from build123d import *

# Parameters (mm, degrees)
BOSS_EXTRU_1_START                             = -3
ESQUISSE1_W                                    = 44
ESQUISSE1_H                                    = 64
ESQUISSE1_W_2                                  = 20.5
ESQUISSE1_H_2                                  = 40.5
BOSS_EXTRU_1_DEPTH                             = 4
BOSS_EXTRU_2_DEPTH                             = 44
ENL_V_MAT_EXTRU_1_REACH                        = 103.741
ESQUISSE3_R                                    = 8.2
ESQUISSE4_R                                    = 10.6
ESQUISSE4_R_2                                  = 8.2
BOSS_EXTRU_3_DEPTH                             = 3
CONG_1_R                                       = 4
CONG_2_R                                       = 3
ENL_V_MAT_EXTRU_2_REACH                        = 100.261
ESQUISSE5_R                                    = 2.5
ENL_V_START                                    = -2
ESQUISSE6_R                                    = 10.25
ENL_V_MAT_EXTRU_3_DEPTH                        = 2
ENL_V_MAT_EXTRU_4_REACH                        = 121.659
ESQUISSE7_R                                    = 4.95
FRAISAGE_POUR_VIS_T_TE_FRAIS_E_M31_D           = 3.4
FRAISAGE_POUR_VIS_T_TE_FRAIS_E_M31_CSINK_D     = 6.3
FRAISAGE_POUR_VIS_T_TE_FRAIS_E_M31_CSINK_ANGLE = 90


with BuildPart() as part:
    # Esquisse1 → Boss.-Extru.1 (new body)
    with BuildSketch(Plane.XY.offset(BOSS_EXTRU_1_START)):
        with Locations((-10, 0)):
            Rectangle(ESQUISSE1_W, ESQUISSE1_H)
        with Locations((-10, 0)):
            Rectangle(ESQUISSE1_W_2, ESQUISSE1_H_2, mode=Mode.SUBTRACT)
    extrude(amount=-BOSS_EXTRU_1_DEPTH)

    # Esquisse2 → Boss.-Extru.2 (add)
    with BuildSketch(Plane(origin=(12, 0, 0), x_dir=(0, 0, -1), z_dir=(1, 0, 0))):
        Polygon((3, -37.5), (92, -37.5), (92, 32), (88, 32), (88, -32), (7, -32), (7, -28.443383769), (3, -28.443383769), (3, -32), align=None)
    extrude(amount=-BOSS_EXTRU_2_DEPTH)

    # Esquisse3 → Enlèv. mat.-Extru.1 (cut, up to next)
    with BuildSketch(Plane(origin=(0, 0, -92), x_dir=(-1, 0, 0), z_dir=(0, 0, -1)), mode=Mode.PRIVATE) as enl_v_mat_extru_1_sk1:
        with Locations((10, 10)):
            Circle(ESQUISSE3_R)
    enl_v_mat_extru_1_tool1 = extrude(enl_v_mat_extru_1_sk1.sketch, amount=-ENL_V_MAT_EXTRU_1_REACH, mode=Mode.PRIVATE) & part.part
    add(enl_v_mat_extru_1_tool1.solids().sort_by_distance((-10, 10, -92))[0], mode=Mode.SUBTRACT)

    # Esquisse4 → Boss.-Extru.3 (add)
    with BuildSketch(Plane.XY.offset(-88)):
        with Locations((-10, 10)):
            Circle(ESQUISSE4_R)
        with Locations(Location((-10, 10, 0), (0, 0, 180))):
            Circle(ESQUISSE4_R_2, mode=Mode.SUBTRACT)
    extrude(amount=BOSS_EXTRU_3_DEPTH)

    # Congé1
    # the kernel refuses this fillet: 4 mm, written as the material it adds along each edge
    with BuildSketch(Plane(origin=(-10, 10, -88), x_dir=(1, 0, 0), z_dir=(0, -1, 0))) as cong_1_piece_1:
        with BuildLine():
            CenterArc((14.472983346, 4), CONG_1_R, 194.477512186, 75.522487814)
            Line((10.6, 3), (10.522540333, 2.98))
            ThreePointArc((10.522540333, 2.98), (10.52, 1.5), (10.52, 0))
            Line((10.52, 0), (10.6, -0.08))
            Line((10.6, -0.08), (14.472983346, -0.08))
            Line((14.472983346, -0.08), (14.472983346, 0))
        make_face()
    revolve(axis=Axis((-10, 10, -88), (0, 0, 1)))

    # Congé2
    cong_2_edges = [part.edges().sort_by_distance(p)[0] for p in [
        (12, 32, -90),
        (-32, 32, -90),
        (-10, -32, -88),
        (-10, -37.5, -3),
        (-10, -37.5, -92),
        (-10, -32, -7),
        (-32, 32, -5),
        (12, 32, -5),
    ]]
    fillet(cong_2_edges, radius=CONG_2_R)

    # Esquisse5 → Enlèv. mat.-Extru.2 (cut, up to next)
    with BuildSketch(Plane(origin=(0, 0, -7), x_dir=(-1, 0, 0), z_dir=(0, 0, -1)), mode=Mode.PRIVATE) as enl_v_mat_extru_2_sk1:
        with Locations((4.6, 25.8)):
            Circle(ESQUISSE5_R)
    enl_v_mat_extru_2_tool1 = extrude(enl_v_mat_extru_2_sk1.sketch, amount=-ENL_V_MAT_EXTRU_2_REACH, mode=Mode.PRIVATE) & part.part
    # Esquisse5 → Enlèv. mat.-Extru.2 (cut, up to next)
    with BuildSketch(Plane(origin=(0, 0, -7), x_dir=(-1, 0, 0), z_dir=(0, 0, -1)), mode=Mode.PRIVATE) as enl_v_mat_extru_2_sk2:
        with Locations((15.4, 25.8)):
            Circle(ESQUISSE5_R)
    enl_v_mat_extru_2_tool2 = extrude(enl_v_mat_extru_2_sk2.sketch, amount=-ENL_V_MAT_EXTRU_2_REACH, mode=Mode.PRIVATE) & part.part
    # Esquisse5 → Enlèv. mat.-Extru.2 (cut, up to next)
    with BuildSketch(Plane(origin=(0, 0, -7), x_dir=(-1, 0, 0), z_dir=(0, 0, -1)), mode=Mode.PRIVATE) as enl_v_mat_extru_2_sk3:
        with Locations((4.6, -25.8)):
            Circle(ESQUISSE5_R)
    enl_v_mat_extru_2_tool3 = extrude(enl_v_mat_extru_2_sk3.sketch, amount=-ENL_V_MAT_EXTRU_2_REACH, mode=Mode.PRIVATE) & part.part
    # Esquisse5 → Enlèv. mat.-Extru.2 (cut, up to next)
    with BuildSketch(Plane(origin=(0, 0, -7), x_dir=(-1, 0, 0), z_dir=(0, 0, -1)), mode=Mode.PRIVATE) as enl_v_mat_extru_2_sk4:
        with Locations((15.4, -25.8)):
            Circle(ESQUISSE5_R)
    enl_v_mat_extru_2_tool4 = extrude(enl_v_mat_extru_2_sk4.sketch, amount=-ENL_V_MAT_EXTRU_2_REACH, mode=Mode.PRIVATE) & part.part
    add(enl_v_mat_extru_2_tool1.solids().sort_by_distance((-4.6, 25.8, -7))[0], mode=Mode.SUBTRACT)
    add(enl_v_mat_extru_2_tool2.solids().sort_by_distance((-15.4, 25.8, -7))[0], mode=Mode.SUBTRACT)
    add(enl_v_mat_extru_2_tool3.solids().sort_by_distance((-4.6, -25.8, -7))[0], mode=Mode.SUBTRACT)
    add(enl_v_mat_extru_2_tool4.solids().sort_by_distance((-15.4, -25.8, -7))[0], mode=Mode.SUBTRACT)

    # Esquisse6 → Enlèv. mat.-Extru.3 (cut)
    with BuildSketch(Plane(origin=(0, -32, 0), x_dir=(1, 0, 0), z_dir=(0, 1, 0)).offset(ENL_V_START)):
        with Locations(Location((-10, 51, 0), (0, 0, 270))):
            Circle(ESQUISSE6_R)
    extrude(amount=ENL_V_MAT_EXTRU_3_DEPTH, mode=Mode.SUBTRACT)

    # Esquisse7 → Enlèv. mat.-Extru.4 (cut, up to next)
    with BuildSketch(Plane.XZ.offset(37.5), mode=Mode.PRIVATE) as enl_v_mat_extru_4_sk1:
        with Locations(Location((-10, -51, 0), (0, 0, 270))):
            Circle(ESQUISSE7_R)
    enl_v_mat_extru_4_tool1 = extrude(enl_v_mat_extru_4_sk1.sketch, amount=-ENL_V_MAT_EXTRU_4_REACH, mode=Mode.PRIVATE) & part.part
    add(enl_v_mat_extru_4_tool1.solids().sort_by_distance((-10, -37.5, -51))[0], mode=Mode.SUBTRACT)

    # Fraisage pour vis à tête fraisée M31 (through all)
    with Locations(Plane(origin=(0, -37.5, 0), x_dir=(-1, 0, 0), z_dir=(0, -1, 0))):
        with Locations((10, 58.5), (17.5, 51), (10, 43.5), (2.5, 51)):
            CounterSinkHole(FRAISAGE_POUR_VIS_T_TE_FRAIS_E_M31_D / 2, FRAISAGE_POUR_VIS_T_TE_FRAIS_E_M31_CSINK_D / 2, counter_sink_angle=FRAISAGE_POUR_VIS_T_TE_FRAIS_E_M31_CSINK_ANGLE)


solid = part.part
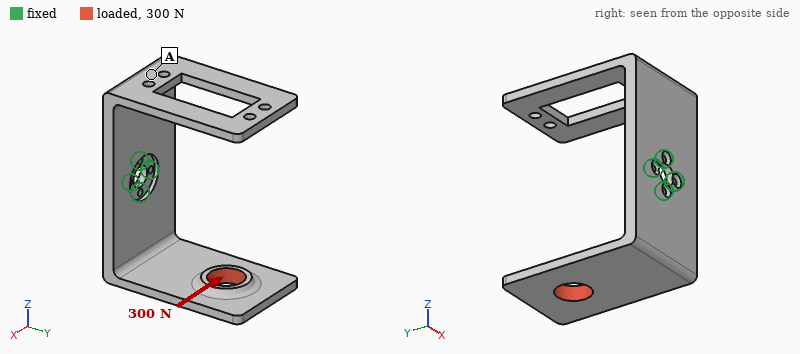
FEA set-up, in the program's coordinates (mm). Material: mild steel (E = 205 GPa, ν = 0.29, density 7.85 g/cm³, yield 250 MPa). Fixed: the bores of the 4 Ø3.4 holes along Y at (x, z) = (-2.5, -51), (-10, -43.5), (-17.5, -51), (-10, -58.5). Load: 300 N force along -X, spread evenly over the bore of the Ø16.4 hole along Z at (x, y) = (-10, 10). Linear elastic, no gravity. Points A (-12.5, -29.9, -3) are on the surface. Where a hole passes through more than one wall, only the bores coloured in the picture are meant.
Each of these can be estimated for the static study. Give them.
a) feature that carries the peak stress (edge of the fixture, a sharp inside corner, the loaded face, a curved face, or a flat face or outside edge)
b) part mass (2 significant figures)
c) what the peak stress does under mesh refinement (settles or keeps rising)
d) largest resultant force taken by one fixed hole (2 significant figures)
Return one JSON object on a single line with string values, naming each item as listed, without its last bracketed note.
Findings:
{"feature that carries the peak stress": "edge of the fixture", "part mass": "310 g", "what the peak stress does under mesh refinement": "keeps rising", "largest resultant force taken by one fixed hole": "670 N"}
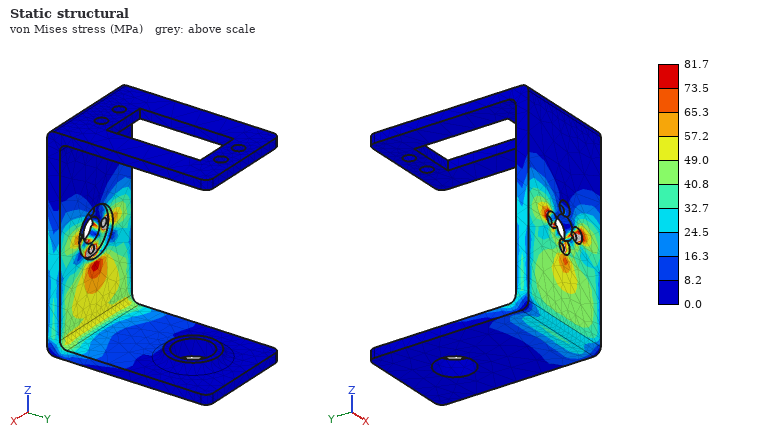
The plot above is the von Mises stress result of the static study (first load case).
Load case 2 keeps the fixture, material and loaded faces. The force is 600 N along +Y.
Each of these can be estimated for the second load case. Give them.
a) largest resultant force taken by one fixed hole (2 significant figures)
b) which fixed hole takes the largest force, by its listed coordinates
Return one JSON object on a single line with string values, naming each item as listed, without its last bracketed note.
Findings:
{"largest resultant force taken by one fixed hole": "1.4 kN", "which fixed hole takes the largest force, by its listed coordinates": "(-10, -58.5)"}
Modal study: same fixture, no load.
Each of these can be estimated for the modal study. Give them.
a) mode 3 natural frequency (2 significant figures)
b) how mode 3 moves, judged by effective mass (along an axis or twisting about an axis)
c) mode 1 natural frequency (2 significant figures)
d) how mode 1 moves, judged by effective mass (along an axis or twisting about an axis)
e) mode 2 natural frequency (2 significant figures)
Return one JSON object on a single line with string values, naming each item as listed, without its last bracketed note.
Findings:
{"mode 3 natural frequency": "860 Hz", "how mode 3 moves, judged by effective mass": "along X", "mode 1 natural frequency": "520 Hz", "how mode 1 moves, judged by effective mass": "along Z", "mode 2 natural frequency": "540 Hz"}
